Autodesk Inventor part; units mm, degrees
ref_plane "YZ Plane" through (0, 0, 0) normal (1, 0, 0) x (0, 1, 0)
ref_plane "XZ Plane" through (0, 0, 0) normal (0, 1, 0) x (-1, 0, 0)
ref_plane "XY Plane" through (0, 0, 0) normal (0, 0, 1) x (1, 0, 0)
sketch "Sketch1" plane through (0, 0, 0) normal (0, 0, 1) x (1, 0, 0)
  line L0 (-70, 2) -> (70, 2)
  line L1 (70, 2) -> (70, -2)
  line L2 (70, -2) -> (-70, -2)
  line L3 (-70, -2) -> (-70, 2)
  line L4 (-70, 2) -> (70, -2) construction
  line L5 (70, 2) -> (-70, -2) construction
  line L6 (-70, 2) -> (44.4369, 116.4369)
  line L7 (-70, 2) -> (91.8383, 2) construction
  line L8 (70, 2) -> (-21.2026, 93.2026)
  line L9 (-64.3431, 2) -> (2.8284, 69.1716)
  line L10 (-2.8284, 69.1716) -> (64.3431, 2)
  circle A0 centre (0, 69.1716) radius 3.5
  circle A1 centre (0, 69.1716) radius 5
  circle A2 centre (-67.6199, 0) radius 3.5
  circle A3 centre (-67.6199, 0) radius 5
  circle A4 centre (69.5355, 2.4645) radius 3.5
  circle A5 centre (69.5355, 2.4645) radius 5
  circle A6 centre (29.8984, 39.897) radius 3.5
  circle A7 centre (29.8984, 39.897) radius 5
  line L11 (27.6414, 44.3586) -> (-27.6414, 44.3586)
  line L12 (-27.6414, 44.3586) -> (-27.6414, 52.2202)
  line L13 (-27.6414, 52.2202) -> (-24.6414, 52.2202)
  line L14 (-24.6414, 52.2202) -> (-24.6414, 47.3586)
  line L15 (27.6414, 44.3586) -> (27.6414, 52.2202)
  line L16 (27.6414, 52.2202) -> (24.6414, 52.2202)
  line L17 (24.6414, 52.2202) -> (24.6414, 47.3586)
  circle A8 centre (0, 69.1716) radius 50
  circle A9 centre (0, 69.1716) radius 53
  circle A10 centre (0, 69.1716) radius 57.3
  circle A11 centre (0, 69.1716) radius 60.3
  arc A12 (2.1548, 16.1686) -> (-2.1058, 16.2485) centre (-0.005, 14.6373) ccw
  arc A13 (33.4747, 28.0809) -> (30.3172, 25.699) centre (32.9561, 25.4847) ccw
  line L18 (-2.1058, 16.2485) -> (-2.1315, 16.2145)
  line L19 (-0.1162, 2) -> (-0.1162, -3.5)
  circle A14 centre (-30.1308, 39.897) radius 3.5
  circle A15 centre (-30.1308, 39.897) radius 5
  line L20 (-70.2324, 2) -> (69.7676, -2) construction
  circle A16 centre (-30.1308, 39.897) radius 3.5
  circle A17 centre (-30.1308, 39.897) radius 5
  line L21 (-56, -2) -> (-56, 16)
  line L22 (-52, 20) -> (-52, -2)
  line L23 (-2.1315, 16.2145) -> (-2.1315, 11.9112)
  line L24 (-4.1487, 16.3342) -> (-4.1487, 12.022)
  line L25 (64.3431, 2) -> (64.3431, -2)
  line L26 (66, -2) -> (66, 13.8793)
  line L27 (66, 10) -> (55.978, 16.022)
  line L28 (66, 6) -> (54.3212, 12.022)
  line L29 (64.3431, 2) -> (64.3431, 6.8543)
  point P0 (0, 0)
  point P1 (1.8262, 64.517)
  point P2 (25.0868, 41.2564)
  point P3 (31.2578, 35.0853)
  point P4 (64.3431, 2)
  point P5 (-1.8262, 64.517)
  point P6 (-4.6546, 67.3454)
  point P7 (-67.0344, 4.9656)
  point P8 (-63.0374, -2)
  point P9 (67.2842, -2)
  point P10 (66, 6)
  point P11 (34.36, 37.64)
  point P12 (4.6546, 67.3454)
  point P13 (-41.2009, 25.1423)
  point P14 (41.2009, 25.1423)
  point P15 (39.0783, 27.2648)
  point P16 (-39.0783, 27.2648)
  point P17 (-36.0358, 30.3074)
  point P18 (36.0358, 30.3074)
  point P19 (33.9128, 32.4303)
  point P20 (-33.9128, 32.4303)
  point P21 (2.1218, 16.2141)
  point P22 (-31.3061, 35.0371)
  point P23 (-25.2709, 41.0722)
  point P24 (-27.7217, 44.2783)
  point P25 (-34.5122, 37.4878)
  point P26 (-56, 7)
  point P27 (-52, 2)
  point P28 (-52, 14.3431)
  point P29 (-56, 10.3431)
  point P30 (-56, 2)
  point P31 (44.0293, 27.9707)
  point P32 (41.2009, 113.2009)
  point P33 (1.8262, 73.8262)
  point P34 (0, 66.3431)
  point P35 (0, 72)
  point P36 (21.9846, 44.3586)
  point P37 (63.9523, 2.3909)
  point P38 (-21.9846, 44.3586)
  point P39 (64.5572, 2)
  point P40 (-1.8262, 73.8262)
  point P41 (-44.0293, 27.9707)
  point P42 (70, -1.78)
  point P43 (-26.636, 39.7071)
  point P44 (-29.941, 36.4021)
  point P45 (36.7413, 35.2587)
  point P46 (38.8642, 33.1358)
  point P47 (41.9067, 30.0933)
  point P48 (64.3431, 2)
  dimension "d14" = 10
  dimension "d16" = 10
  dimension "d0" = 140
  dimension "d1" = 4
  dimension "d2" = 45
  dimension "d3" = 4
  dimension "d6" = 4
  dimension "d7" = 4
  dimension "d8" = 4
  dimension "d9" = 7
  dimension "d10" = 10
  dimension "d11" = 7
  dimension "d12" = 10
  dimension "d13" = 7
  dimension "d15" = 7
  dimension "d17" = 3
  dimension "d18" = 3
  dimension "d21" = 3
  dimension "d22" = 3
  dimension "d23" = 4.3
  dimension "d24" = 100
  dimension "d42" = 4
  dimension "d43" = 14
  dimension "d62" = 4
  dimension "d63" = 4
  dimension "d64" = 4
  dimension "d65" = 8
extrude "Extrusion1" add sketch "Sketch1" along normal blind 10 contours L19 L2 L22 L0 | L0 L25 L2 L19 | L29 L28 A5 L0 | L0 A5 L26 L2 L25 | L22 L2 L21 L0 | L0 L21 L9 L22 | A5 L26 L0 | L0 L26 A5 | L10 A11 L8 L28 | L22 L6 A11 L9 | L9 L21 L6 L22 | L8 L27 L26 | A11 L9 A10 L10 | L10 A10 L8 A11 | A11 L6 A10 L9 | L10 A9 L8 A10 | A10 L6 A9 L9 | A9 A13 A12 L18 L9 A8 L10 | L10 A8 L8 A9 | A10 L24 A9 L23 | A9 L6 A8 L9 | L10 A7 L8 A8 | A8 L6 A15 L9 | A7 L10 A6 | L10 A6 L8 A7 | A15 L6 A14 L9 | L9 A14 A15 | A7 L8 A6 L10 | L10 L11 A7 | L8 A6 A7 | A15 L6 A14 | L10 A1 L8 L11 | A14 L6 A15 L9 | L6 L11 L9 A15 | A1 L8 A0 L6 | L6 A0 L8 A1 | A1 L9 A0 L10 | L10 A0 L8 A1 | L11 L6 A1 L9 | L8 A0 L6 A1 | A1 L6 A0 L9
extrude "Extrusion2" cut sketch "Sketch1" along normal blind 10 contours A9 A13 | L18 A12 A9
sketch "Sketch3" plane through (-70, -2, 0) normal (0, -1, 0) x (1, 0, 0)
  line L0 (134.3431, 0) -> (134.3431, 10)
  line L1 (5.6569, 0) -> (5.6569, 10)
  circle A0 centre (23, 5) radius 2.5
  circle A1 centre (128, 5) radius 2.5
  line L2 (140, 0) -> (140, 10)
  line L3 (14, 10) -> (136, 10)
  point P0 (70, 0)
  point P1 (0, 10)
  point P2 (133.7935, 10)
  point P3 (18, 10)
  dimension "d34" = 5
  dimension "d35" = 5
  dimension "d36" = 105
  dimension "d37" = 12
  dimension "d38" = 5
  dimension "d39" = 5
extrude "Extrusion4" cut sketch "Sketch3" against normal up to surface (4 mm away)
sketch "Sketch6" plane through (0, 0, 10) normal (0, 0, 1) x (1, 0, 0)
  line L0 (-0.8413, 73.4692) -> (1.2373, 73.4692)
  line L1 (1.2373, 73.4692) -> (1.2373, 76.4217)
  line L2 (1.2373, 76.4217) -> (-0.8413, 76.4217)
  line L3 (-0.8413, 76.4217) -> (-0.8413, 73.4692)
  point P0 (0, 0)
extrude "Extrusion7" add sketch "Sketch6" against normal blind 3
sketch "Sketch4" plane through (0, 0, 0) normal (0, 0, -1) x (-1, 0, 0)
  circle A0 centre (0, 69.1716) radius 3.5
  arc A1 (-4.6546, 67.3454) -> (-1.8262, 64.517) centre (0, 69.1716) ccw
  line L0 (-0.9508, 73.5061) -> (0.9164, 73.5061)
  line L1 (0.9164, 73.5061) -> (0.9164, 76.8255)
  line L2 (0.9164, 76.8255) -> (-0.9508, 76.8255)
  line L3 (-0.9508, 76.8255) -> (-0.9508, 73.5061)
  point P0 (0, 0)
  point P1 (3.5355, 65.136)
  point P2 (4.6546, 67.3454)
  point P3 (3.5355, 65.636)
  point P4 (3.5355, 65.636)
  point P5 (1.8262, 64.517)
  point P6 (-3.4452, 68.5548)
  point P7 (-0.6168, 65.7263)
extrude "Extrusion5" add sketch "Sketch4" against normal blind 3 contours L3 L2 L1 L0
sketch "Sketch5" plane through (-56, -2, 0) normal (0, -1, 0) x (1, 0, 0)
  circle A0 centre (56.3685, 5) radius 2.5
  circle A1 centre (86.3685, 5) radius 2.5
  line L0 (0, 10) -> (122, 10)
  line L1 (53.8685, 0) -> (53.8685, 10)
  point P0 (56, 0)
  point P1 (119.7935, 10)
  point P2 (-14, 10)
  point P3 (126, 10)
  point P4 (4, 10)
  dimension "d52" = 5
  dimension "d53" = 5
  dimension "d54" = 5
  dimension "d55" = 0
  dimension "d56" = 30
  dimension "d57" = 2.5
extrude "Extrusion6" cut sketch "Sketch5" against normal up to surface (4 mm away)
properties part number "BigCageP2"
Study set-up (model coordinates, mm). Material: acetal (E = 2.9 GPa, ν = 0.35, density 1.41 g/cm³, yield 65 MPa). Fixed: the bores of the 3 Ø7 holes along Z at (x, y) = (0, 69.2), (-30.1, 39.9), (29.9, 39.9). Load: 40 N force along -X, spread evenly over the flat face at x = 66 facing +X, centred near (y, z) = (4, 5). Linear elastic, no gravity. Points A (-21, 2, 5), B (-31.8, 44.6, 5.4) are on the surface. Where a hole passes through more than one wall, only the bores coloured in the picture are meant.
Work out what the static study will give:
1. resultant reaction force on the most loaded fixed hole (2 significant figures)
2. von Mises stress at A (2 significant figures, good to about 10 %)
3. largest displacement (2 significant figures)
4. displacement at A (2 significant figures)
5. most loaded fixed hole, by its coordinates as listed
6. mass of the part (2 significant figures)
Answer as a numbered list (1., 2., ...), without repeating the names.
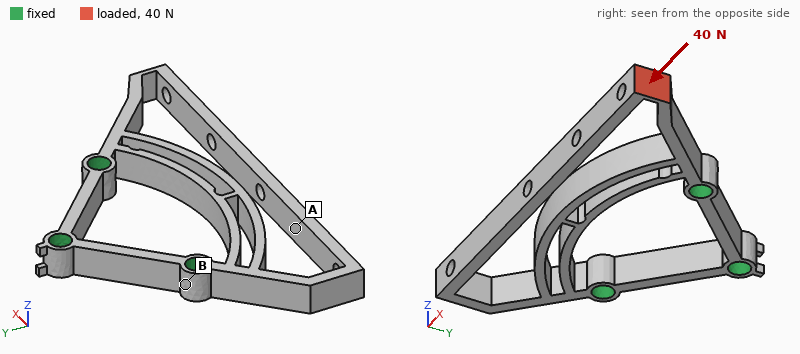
1. 24 N
2. 3.5 MPa
3. 1.7 mm
4. 1.3 mm
5. (29.9, 39.9)
6. 24 g
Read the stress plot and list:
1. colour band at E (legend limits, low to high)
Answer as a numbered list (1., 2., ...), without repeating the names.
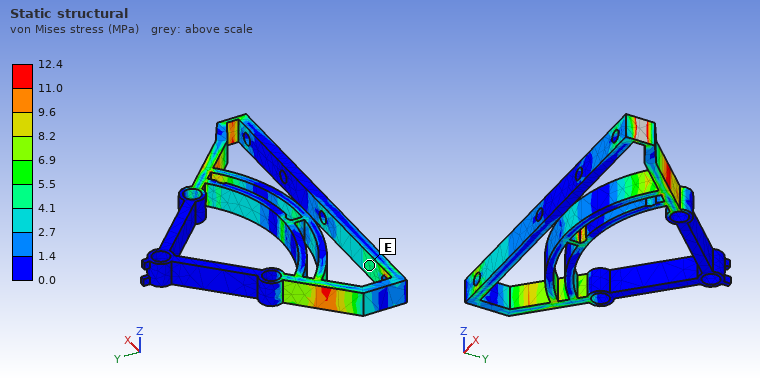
1. 4.1 to 5.5 MPa
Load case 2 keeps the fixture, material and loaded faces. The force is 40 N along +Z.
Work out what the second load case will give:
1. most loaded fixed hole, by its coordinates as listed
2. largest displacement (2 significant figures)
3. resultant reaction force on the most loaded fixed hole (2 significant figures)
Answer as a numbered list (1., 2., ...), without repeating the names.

1. (29.9, 39.9)
2. 1.6 mm
3. 42 N
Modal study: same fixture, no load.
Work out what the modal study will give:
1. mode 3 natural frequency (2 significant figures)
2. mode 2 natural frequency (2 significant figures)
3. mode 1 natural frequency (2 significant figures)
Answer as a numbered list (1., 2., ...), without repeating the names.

1. 320 Hz
2. 320 Hz
3. 230 Hz
